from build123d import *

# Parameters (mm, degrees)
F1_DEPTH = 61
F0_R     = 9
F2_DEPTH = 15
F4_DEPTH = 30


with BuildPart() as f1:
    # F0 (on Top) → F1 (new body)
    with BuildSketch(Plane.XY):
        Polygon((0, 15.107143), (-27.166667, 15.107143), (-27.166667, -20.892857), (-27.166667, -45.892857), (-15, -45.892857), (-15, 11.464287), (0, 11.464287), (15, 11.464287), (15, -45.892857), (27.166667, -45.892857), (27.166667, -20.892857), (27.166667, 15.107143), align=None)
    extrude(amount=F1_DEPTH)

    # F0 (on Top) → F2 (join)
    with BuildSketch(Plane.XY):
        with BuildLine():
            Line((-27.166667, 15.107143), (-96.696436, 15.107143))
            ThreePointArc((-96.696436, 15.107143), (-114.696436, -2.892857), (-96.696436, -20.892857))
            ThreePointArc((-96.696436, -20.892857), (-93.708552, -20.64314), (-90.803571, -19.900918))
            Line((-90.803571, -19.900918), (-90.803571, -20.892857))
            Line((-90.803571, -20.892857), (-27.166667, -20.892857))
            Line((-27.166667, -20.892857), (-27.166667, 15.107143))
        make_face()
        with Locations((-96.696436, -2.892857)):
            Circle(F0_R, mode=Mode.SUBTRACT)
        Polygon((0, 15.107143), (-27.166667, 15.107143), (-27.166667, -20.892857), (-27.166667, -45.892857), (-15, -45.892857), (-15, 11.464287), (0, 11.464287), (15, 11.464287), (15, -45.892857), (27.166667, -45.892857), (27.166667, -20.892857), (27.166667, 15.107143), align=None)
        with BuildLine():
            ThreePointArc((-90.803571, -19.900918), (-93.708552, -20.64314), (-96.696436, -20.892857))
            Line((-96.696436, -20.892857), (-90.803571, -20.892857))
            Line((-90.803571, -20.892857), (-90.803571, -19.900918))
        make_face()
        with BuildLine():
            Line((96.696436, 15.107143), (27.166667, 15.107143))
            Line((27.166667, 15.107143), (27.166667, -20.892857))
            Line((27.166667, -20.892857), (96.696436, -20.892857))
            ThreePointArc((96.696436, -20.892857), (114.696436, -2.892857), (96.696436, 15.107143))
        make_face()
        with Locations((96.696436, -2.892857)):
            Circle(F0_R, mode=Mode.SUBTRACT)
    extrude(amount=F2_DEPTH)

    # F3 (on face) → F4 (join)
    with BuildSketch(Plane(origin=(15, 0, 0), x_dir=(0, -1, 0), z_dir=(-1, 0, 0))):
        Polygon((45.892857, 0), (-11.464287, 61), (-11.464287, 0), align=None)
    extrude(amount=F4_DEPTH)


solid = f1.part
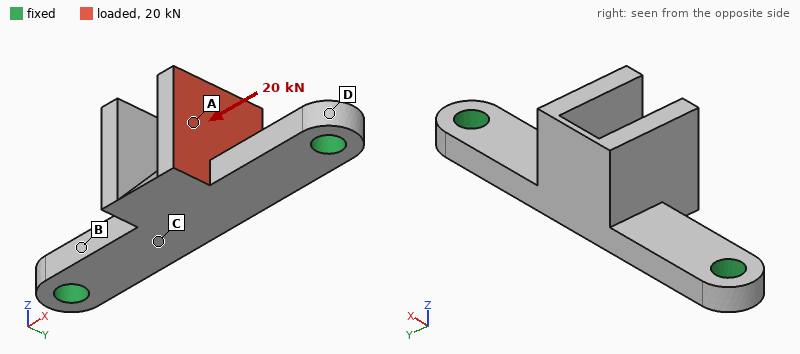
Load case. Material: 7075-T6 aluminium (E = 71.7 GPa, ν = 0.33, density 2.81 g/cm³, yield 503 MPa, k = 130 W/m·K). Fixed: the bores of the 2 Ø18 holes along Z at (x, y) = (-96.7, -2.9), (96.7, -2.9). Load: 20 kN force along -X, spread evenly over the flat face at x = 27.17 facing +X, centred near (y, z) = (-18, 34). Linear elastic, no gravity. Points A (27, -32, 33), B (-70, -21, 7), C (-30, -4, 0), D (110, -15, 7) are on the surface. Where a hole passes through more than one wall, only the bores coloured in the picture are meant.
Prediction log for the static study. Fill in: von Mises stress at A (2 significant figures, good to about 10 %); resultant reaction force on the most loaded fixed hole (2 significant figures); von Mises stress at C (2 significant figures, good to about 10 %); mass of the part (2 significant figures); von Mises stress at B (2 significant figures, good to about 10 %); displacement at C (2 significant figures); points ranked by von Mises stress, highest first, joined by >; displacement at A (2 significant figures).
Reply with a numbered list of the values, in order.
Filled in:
1. 47 MPa
2. 11 kN
3. 69 MPa
4. 650 g
5. 32 MPa
6. 0.089 mm
7. C > A > B > D
8. 0.20 mm
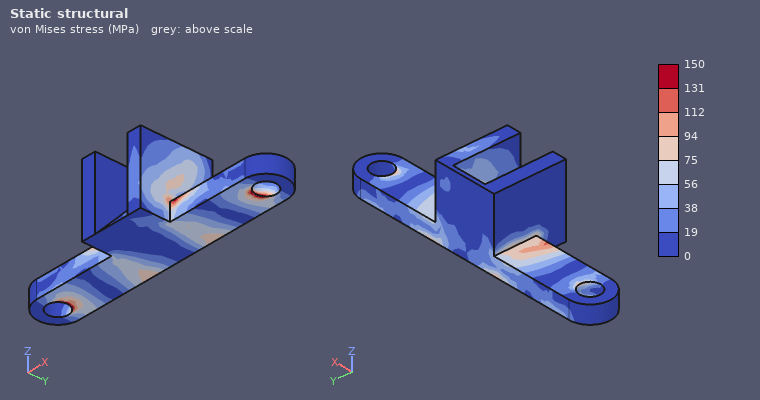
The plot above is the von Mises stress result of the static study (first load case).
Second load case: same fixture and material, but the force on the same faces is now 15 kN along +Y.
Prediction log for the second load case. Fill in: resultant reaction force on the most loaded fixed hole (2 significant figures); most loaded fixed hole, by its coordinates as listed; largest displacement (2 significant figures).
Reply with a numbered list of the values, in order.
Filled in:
1. 10 kN
2. (96.7, -2.9)
3. 1.2 mm
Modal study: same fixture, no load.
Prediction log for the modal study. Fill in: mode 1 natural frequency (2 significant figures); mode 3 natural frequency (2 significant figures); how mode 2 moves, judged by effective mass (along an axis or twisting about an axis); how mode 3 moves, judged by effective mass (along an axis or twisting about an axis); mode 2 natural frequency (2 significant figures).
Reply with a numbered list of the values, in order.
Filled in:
1. 1100 Hz
2. 2800 Hz
3. along Z
4. along X
5. 1600 Hz
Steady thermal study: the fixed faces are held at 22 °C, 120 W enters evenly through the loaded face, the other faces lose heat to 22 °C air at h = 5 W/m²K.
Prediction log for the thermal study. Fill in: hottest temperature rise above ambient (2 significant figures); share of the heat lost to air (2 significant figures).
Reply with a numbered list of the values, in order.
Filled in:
1. 83 K
2. 6.2 %
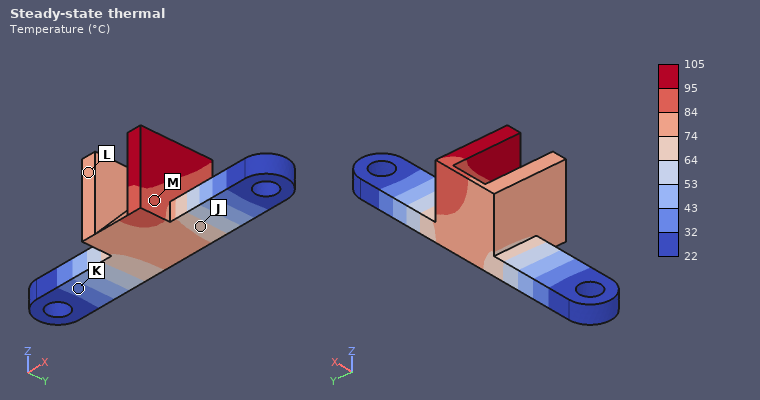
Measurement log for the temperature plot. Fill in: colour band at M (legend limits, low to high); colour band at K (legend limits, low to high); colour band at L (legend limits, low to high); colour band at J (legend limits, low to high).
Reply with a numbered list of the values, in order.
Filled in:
1. 84 to 95 °C
2. 32 to 43 °C
3. 74 to 84 °C
4. 64 to 74 °C
